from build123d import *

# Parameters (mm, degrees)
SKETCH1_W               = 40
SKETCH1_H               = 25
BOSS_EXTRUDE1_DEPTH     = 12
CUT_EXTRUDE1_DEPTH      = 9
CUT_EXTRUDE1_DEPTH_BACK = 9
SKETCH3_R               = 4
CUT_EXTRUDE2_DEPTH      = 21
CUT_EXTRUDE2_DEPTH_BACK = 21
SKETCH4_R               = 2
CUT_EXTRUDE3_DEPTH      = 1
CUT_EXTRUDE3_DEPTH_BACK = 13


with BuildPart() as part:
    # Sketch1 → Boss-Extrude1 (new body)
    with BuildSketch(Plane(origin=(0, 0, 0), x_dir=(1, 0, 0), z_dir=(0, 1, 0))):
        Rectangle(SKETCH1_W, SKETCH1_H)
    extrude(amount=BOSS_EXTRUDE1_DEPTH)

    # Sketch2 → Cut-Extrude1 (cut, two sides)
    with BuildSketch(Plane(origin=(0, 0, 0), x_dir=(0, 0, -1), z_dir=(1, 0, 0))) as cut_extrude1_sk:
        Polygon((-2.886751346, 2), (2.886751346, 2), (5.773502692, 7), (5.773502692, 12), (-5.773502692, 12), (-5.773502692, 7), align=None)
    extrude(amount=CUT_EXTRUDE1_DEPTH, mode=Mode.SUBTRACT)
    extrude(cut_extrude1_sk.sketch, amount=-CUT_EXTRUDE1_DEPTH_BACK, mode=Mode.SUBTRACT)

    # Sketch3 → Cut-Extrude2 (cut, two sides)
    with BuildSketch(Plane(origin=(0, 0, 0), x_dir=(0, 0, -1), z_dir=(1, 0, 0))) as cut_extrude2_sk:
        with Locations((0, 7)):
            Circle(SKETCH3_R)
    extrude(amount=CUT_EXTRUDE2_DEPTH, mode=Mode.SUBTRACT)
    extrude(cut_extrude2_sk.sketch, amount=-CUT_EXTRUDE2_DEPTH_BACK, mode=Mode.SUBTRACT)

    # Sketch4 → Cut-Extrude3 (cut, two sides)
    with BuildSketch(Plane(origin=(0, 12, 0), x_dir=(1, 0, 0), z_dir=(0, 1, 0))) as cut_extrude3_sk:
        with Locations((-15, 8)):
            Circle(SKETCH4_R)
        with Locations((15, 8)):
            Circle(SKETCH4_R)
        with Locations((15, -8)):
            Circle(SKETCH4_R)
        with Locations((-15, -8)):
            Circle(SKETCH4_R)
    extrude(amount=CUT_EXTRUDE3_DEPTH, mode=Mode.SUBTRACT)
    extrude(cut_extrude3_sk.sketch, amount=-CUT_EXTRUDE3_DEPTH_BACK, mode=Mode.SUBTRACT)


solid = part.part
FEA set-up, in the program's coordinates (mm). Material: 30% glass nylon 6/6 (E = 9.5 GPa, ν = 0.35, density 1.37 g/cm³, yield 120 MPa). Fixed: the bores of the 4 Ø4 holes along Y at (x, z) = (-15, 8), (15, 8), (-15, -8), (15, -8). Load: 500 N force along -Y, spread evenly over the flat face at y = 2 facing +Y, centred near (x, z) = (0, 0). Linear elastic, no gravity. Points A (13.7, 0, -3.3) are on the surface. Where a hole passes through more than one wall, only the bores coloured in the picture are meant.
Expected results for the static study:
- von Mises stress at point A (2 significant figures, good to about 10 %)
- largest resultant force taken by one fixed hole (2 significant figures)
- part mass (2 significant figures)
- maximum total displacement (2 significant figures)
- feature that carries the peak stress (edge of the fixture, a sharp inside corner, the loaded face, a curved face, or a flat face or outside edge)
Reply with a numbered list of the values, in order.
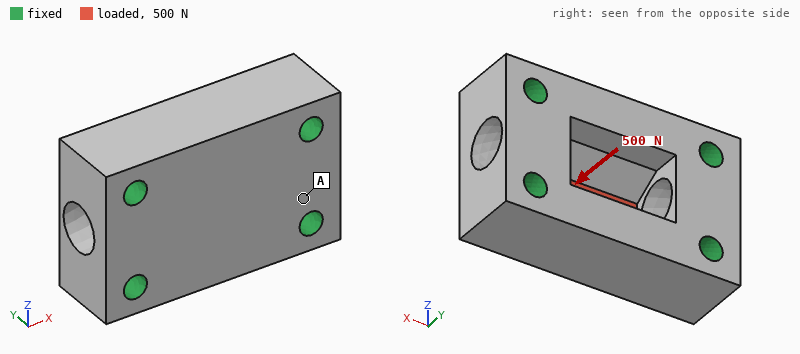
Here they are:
1. 3.0 MPa
2. 140 N
3. 12 g
4. 25 µm
5. a flat face or outside edge
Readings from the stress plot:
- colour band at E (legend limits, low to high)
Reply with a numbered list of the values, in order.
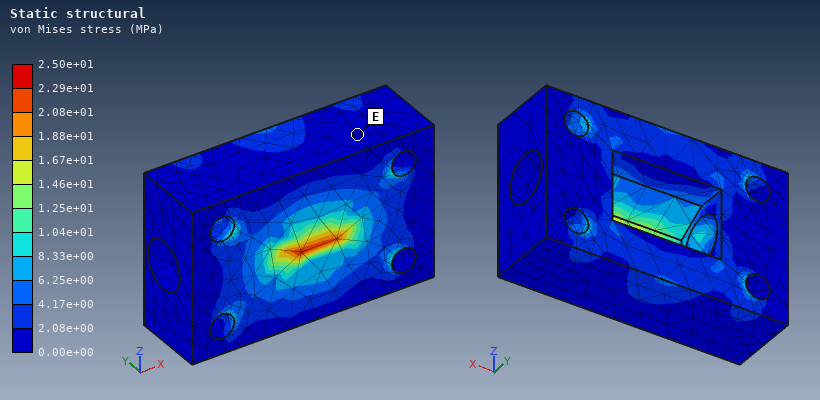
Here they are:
1. 0.00e+00 to 2.08e+00 MPa
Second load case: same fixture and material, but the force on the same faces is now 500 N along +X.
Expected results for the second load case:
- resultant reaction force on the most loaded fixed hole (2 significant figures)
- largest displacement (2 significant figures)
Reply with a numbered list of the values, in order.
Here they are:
1. 130 N
2. 8.3 µm
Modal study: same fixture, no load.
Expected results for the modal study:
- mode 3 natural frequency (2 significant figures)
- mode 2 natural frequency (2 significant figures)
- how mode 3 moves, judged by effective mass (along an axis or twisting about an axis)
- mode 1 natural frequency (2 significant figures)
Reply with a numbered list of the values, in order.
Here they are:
1. 23 kHz
2. 22 kHz
3. along Y
4. 21 kHz
